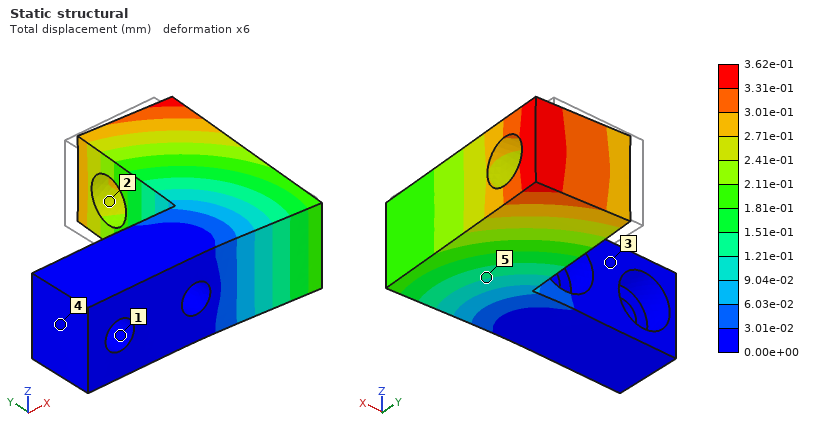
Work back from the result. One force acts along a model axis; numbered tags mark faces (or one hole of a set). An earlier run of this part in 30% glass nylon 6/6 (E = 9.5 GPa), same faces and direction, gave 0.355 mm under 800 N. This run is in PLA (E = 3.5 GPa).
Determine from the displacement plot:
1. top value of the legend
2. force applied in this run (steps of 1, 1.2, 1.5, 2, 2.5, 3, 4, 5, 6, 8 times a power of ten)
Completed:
3.62e-01 mm
300 N
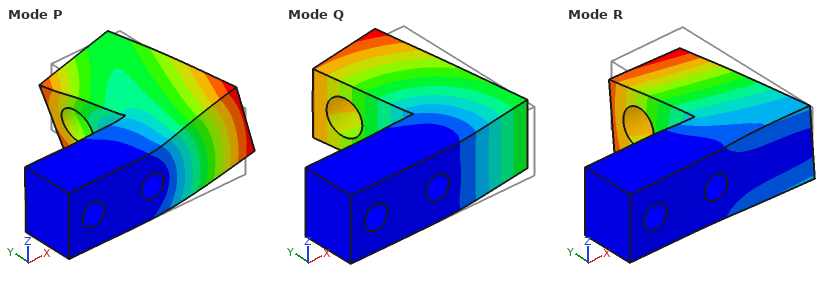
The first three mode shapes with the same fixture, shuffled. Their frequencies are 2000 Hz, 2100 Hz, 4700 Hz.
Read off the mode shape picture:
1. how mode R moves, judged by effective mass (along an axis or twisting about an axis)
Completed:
along Z
